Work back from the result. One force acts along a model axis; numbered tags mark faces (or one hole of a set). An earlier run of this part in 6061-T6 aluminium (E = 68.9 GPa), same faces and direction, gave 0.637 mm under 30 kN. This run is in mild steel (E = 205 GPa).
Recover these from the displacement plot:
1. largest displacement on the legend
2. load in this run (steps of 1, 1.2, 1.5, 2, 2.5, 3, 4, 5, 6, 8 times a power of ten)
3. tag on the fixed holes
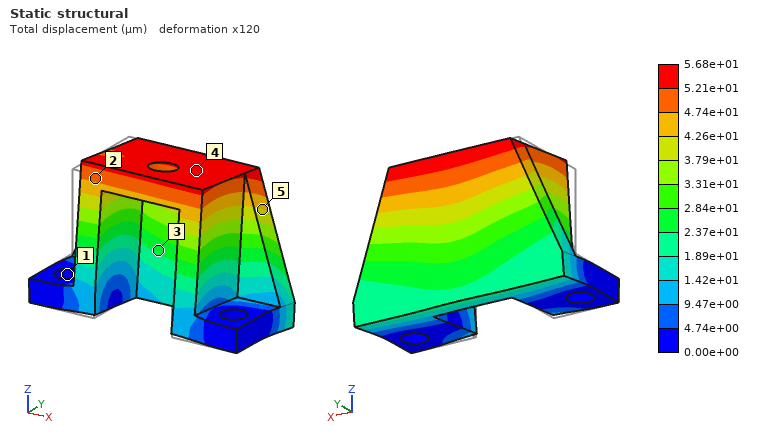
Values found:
5.68e+01 µm
8 kN
1
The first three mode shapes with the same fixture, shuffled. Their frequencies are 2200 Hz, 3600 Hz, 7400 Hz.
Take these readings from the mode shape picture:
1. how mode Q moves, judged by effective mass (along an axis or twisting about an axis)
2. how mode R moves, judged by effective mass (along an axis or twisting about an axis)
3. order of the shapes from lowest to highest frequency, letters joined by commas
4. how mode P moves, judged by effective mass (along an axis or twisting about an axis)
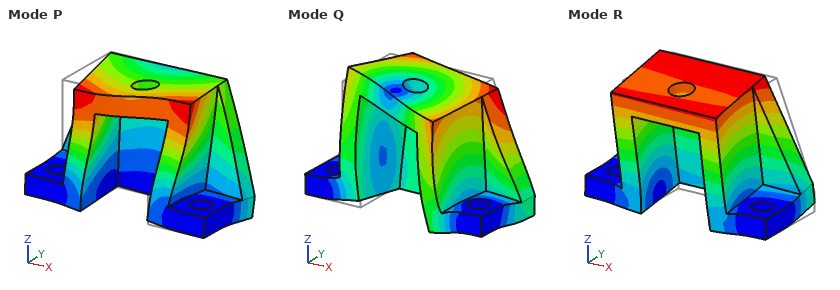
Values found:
along X
along Y
R, P, Q
along X
